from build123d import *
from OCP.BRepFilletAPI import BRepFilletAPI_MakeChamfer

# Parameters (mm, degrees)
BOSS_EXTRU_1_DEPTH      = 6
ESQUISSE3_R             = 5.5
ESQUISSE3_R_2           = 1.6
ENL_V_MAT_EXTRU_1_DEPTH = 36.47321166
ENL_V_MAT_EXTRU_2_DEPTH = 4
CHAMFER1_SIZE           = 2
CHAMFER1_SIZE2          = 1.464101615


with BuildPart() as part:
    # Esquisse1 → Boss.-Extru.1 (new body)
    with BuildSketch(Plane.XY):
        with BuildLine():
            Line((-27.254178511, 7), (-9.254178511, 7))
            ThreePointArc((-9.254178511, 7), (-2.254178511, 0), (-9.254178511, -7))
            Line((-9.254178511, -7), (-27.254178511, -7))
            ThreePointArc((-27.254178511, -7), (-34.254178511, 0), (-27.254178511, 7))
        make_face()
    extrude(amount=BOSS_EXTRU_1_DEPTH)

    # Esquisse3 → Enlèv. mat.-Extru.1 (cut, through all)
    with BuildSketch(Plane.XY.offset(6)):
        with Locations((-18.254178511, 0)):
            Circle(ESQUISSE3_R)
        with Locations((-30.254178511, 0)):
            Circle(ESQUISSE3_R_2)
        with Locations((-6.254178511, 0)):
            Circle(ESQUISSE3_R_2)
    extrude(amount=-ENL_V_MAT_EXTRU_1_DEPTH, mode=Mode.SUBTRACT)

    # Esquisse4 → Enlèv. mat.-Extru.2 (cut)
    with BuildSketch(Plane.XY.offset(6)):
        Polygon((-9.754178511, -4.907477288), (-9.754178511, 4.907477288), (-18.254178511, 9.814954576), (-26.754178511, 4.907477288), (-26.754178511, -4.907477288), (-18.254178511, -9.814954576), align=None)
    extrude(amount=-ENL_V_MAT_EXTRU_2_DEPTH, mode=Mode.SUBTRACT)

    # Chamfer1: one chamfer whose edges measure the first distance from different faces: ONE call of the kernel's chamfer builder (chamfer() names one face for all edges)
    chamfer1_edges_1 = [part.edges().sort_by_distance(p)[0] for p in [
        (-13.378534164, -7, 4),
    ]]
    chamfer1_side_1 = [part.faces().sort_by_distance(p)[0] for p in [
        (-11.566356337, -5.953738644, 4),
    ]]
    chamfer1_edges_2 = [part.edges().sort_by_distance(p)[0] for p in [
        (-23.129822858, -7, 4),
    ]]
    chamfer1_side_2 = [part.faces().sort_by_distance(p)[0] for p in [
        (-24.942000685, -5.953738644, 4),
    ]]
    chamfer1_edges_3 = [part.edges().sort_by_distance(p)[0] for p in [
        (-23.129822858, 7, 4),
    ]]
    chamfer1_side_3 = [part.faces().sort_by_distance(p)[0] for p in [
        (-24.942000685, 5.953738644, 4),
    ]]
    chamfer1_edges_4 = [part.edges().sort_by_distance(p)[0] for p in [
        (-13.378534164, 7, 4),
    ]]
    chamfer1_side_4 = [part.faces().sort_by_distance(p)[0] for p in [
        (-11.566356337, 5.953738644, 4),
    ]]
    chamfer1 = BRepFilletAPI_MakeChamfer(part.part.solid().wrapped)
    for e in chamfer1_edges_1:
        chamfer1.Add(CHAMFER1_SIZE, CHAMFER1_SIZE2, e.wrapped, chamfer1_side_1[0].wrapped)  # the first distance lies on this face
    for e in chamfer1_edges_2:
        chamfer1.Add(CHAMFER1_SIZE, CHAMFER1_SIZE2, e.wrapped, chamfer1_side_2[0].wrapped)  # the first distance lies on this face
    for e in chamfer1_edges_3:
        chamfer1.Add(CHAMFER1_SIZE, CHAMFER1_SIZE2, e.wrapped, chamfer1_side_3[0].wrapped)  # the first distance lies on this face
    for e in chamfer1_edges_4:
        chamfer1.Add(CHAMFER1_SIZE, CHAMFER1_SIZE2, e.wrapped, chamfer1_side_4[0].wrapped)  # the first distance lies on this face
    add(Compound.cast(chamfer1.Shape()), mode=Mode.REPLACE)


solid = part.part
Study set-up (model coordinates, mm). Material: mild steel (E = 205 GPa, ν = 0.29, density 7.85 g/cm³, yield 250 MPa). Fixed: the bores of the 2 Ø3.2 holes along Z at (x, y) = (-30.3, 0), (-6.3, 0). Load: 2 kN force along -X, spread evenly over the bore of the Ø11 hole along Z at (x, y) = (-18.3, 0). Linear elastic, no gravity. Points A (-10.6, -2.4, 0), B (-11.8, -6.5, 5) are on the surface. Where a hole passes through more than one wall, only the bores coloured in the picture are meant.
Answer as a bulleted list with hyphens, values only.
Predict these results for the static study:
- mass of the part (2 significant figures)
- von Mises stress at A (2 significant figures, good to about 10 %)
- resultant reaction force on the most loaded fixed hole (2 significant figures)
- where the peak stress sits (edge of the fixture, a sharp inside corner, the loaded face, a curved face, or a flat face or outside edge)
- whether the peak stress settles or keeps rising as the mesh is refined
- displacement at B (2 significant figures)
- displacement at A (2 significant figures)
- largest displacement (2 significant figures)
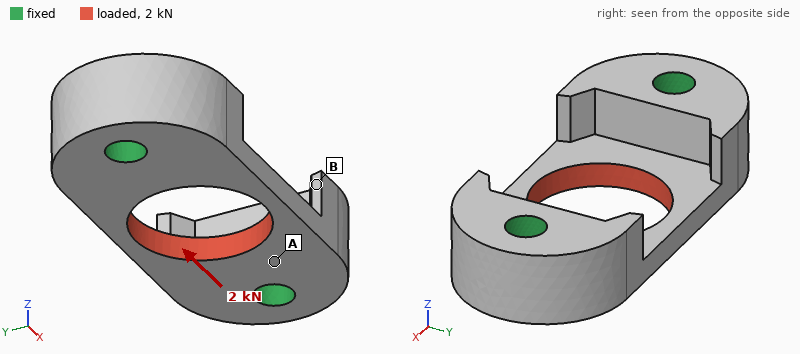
- 9.8 g
- 41 MPa
- 1.0 kN
- edge of the fixture
- keeps rising
- 1.1 µm
- 1.2 µm
- 3.2 µm
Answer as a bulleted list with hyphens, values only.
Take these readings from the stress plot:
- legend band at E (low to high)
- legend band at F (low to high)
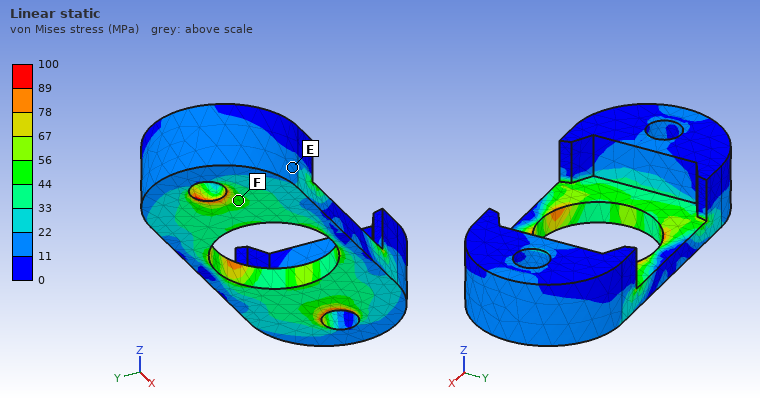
- 11 to 22 MPa
- 44 to 56 MPa
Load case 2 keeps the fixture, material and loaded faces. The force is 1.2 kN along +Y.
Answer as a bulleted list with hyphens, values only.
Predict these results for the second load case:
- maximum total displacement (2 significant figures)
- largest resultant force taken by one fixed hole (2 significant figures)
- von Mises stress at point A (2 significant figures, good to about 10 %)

- 6.5 µm
- 600 N
- 49 MPa
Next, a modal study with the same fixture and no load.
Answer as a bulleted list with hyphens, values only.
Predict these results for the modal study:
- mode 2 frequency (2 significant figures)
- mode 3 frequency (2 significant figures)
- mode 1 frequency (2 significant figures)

- 39 kHz
- 56 kHz
- 39 kHz
